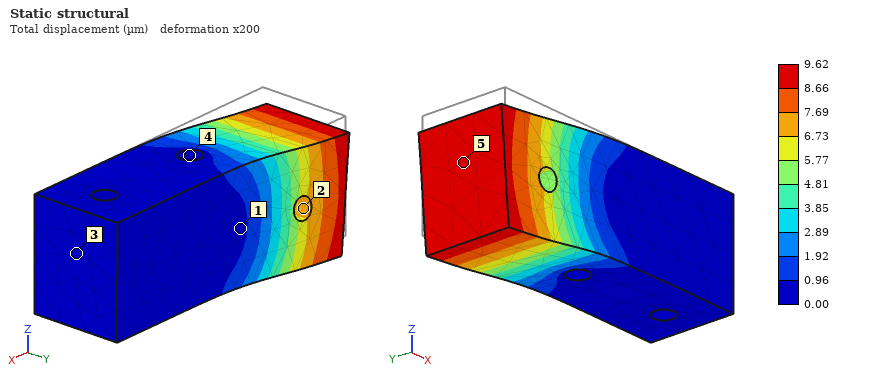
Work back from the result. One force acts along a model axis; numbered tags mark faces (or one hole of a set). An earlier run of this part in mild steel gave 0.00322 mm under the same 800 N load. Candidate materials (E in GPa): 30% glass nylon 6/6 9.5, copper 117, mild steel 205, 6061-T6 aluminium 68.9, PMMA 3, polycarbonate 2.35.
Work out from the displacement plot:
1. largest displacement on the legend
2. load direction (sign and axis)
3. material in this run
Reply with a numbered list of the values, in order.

1. 9.62 µm
2. -Z
3. 6061-T6 aluminium
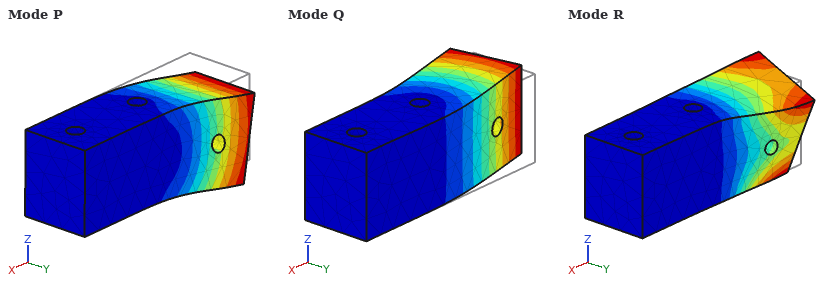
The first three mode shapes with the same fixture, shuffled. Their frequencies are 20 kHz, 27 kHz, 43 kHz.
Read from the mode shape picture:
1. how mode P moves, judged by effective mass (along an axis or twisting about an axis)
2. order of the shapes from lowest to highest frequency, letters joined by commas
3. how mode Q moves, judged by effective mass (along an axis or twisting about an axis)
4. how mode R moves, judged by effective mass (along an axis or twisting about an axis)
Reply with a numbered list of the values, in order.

1. along Z
2. Q, P, R
3. along Y
4. twisting about X
